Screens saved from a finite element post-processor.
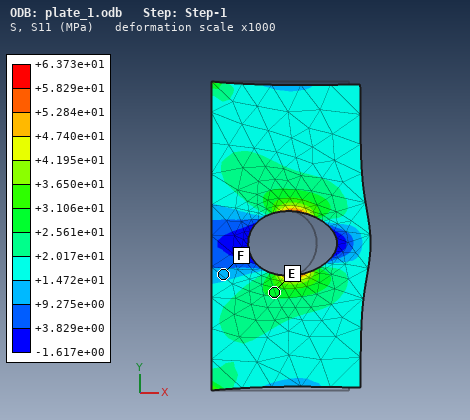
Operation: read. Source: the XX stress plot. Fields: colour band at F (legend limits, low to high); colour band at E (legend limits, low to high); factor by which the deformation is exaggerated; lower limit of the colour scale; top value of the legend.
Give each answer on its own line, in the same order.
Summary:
+9.275e+00 to +1.472e+01 MPa
+2.561e+01 to +3.106e+01 MPa
1000
-1.617e+00 MPa
+6.373e+01 MPa
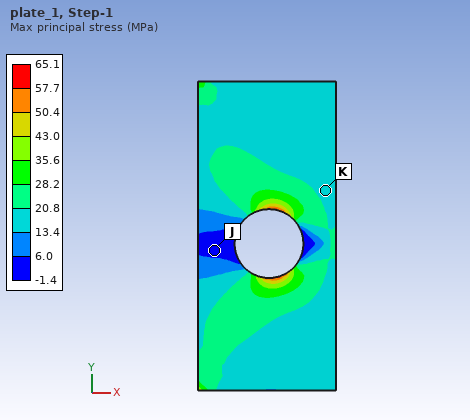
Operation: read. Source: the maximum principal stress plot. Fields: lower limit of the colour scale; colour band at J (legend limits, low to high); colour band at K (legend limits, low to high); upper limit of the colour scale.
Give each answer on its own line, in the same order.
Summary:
-1.4 MPa
-1.4 to 6.0 MPa
13.4 to 20.8 MPa
65.1 MPa
